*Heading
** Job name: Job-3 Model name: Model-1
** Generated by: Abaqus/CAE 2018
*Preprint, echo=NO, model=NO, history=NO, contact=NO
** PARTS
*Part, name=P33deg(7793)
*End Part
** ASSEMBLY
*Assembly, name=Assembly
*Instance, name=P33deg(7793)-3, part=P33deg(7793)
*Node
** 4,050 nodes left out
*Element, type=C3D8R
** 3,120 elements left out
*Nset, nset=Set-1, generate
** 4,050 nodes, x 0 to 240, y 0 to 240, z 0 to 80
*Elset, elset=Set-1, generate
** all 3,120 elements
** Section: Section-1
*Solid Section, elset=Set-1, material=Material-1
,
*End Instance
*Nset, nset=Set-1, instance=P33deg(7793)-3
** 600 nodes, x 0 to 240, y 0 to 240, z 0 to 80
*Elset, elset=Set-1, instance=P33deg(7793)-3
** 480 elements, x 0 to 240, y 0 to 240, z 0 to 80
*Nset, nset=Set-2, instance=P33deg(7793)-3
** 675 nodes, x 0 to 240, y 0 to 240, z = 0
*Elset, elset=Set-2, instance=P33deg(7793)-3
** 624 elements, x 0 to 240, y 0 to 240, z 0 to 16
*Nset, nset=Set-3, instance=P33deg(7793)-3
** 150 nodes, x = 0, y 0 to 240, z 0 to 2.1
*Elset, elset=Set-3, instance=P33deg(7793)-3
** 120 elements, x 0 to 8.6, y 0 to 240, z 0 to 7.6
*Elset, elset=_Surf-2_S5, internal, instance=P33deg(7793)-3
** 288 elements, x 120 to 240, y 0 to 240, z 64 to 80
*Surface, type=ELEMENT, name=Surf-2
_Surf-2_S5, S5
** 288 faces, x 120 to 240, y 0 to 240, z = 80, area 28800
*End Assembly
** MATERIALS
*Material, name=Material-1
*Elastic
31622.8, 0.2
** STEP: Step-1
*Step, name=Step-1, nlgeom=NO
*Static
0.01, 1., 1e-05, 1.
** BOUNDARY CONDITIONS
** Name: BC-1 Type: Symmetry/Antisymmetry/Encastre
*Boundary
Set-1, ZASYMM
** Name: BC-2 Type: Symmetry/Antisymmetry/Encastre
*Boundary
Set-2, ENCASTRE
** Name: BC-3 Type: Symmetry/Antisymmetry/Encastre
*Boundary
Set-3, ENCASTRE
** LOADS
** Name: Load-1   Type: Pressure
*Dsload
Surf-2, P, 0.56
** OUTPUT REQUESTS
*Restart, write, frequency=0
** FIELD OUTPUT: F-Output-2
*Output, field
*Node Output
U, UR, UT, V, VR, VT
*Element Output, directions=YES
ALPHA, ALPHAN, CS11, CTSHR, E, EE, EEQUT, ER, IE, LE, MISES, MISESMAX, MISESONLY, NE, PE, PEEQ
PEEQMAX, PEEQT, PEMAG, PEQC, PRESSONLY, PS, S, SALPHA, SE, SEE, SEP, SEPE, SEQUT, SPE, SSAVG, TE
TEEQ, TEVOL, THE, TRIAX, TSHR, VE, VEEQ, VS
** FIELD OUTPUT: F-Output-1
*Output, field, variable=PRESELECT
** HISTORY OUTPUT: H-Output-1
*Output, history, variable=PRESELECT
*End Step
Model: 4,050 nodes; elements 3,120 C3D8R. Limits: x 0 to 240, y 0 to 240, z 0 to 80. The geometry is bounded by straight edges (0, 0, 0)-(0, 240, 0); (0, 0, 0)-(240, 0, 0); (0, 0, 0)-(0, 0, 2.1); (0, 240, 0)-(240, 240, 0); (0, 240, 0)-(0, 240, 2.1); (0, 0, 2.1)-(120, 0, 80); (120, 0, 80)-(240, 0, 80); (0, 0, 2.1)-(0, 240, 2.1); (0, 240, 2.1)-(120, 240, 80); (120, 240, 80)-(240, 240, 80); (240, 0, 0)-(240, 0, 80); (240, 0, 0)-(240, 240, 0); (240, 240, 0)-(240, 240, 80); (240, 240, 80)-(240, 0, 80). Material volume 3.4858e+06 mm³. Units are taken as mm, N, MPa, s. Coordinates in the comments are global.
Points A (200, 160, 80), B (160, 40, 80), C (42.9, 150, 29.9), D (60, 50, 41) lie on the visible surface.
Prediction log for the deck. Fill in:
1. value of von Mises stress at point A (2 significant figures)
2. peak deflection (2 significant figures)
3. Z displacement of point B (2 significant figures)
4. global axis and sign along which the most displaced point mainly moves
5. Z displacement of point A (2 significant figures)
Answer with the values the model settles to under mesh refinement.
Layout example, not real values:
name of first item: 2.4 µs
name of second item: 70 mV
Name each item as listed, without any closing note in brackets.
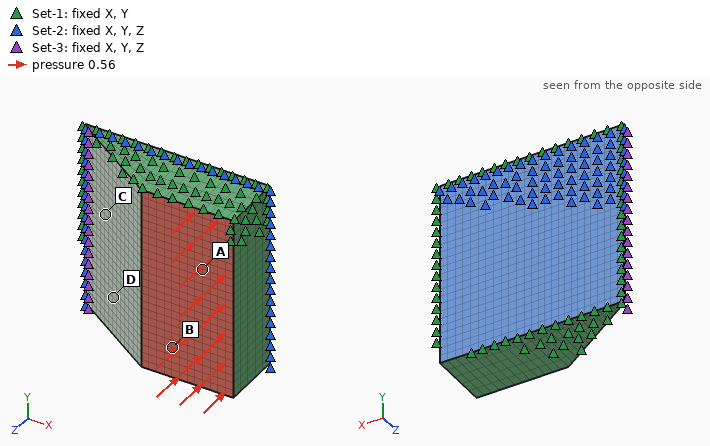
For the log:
value of von Mises stress at point A: 0.40 MPa
peak deflection: 0.0013 mm
Z displacement of point B: -0.0012 mm
global axis and sign along which the most displaced point mainly moves: -Z
Z displacement of point A: -0.0013 mm
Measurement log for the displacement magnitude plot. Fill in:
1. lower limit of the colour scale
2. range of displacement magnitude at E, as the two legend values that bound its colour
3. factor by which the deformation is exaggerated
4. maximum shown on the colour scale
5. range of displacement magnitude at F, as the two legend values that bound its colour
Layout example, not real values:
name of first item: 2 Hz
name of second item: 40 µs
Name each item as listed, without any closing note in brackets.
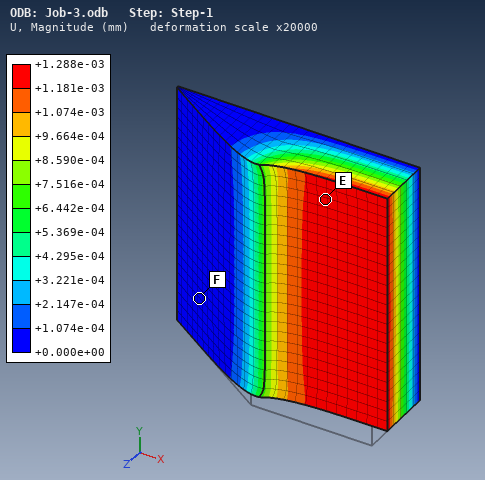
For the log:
lower limit of the colour scale: +0.000e+00 mm
range of displacement magnitude at E, as the two legend values that bound its colour: +1.181e-03 to +1.288e-03 mm
factor by which the deformation is exaggerated: 20000
maximum shown on the colour scale: +1.288e-03 mm
range of displacement magnitude at F, as the two legend values that bound its colour: +0.000e+00 to +1.074e-04 mm
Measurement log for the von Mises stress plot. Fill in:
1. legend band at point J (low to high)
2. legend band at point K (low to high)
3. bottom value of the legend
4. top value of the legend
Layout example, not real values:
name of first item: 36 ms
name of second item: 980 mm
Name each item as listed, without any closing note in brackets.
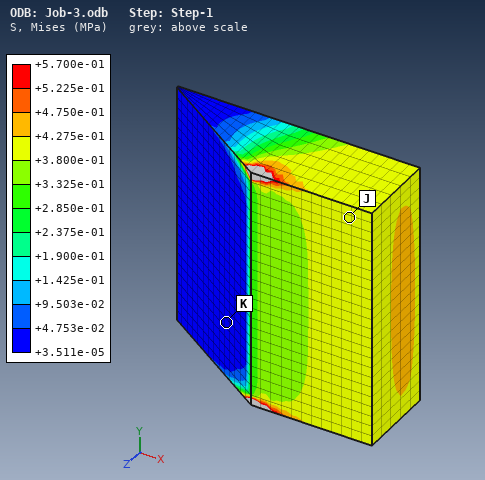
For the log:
legend band at point J: +3.800e-01 to +4.275e-01 MPa
legend band at point K: +3.511e-05 to +4.753e-02 MPa
bottom value of the legend: +3.511e-05 MPa
top value of the legend: +5.700e-01 MPa
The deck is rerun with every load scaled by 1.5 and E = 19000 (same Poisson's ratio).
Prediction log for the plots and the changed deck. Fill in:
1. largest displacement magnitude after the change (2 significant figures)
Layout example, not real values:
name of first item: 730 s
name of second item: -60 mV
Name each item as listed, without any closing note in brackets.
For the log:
largest displacement magnitude after the change: 0.0032 mm
